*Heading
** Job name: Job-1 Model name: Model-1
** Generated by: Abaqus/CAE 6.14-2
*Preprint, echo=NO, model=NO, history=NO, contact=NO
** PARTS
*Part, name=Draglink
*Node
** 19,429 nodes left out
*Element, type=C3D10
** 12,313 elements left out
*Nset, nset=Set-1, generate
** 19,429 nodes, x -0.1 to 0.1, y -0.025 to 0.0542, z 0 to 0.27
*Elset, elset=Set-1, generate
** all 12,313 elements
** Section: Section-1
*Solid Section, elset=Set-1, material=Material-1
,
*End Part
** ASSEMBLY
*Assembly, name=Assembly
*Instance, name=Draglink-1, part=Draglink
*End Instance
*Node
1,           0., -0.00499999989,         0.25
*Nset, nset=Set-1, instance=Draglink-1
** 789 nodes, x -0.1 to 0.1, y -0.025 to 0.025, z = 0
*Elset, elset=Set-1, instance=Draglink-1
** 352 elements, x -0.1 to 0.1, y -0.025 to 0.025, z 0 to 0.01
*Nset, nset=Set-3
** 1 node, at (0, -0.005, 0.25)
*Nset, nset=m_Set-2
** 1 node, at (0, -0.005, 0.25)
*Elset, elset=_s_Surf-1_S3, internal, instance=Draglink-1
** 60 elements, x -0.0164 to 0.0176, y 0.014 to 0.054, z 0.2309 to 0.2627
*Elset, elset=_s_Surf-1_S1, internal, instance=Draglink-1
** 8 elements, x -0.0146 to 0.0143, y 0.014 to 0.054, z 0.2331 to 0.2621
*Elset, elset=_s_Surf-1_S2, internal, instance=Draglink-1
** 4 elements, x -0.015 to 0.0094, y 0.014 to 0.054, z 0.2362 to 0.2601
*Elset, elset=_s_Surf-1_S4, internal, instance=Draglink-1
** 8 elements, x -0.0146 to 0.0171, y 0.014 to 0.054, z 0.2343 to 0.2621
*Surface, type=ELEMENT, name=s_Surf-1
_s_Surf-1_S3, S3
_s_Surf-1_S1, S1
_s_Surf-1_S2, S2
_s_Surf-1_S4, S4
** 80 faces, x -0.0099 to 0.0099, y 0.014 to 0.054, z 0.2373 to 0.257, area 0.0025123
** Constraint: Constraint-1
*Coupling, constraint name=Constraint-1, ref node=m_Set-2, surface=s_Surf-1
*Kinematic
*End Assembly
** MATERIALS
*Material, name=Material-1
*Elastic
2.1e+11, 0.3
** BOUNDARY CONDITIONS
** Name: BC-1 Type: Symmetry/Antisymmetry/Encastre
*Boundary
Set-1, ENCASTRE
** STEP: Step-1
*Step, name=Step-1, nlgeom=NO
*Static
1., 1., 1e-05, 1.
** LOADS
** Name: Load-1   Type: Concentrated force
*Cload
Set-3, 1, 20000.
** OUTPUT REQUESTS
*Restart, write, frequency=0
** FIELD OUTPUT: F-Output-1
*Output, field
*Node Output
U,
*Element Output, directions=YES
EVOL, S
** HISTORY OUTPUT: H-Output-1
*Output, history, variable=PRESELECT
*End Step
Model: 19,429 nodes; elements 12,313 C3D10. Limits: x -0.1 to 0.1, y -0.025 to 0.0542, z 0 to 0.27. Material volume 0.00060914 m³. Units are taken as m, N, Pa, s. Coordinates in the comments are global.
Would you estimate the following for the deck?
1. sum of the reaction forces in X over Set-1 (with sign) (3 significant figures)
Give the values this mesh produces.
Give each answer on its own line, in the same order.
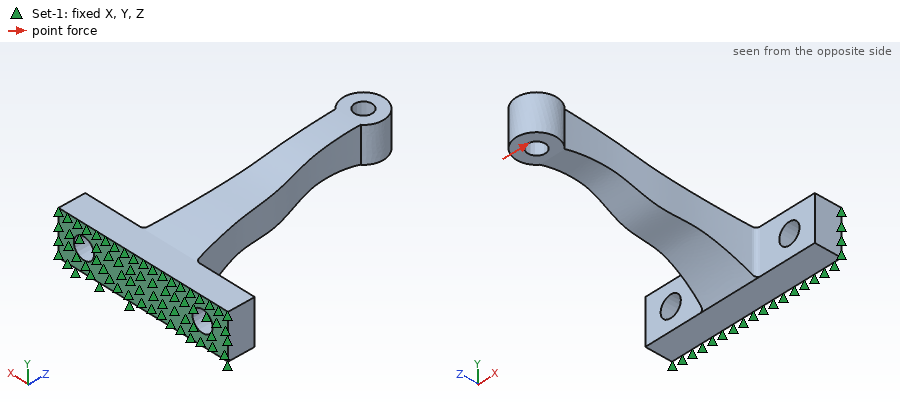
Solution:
-20000 N
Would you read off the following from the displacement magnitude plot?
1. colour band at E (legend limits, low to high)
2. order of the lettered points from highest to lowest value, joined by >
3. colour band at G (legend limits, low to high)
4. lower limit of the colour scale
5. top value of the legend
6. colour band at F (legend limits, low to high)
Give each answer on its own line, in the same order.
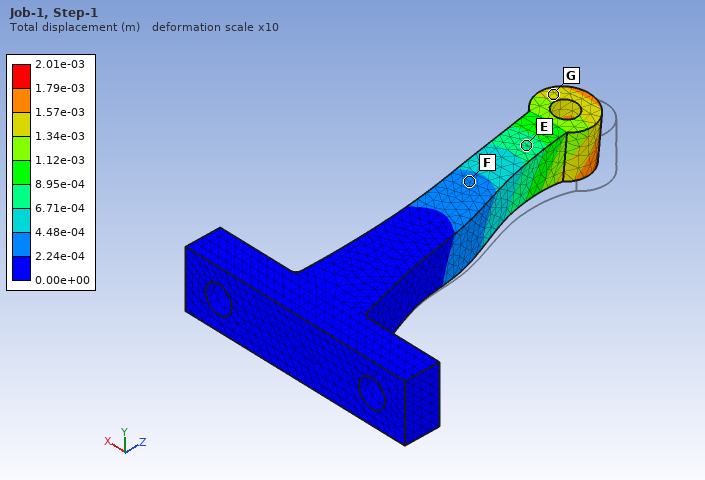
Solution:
6.71e-04 to 8.95e-04 m
G > E > F
1.34e-03 to 1.57e-03 m
0.00e+00 m
2.01e-03 m
2.24e-04 to 4.48e-04 m
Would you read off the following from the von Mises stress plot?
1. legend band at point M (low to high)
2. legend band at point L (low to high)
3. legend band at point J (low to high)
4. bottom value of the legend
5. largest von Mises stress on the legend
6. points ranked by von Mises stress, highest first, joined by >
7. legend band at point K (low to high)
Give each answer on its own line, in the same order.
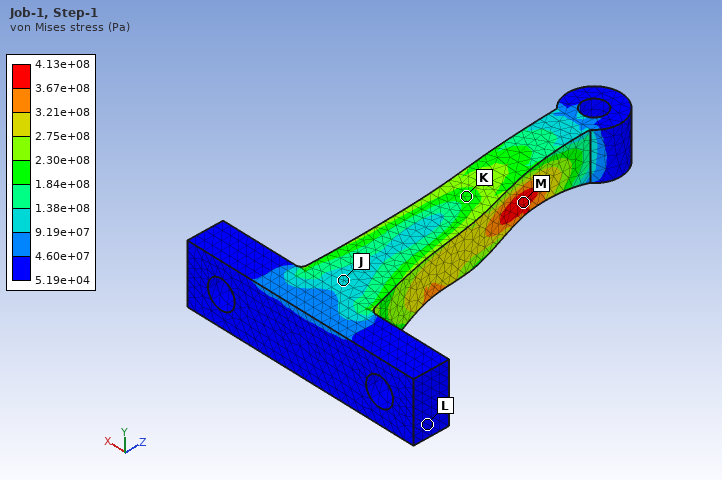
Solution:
3.67e+08 to 4.13e+08 Pa
5.19e+04 to 4.60e+07 Pa
9.19e+07 to 1.38e+08 Pa
5.19e+04 Pa
4.13e+08 Pa
M > K > J > L
1.84e+08 to 2.30e+08 Pa
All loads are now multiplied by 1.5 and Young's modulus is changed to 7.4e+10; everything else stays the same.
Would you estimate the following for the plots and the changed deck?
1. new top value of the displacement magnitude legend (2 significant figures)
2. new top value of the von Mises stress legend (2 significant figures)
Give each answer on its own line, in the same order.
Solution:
0.0086 m
6.2e+08 Pa
